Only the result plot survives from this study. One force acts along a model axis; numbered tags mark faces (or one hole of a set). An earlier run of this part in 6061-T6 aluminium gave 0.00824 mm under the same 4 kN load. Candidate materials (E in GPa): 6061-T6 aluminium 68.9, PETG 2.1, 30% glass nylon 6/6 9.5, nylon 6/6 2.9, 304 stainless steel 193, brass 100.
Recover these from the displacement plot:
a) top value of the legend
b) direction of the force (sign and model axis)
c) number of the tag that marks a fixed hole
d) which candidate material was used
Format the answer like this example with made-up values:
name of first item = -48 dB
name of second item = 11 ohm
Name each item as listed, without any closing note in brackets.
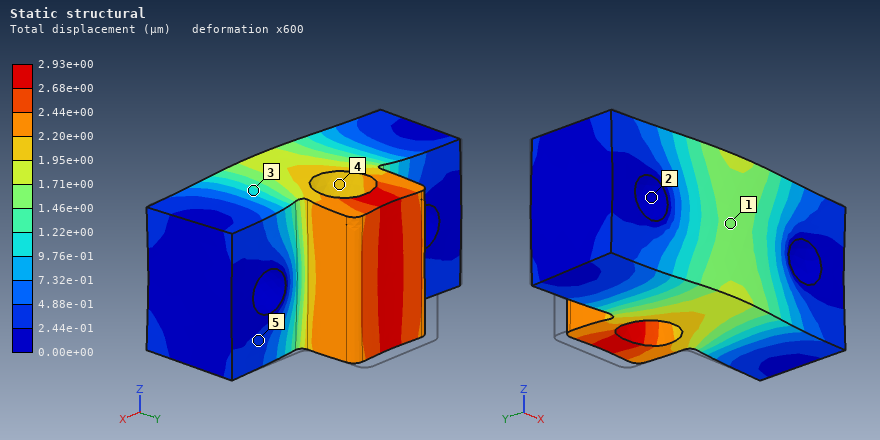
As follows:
top value of the legend = 2.93e+00 µm
direction of the force = -Y
number of the tag that marks a fixed hole = 2
which candidate material was used = 304 stainless steel
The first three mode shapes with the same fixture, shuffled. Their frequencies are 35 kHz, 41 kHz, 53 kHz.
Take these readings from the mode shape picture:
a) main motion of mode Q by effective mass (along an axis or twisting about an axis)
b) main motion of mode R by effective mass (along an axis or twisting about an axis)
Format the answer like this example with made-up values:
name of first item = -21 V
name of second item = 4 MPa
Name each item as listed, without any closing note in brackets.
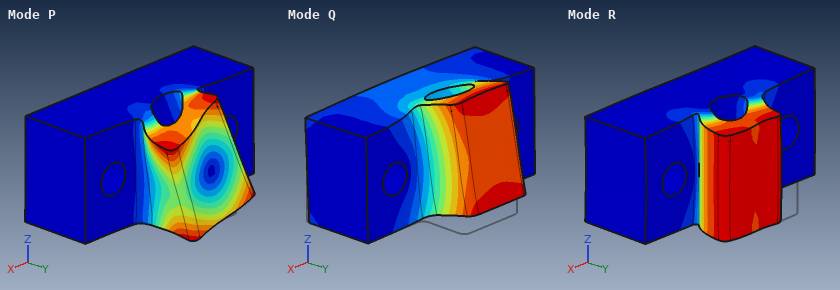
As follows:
main motion of mode Q by effective mass = along Z
main motion of mode R by effective mass = along X
